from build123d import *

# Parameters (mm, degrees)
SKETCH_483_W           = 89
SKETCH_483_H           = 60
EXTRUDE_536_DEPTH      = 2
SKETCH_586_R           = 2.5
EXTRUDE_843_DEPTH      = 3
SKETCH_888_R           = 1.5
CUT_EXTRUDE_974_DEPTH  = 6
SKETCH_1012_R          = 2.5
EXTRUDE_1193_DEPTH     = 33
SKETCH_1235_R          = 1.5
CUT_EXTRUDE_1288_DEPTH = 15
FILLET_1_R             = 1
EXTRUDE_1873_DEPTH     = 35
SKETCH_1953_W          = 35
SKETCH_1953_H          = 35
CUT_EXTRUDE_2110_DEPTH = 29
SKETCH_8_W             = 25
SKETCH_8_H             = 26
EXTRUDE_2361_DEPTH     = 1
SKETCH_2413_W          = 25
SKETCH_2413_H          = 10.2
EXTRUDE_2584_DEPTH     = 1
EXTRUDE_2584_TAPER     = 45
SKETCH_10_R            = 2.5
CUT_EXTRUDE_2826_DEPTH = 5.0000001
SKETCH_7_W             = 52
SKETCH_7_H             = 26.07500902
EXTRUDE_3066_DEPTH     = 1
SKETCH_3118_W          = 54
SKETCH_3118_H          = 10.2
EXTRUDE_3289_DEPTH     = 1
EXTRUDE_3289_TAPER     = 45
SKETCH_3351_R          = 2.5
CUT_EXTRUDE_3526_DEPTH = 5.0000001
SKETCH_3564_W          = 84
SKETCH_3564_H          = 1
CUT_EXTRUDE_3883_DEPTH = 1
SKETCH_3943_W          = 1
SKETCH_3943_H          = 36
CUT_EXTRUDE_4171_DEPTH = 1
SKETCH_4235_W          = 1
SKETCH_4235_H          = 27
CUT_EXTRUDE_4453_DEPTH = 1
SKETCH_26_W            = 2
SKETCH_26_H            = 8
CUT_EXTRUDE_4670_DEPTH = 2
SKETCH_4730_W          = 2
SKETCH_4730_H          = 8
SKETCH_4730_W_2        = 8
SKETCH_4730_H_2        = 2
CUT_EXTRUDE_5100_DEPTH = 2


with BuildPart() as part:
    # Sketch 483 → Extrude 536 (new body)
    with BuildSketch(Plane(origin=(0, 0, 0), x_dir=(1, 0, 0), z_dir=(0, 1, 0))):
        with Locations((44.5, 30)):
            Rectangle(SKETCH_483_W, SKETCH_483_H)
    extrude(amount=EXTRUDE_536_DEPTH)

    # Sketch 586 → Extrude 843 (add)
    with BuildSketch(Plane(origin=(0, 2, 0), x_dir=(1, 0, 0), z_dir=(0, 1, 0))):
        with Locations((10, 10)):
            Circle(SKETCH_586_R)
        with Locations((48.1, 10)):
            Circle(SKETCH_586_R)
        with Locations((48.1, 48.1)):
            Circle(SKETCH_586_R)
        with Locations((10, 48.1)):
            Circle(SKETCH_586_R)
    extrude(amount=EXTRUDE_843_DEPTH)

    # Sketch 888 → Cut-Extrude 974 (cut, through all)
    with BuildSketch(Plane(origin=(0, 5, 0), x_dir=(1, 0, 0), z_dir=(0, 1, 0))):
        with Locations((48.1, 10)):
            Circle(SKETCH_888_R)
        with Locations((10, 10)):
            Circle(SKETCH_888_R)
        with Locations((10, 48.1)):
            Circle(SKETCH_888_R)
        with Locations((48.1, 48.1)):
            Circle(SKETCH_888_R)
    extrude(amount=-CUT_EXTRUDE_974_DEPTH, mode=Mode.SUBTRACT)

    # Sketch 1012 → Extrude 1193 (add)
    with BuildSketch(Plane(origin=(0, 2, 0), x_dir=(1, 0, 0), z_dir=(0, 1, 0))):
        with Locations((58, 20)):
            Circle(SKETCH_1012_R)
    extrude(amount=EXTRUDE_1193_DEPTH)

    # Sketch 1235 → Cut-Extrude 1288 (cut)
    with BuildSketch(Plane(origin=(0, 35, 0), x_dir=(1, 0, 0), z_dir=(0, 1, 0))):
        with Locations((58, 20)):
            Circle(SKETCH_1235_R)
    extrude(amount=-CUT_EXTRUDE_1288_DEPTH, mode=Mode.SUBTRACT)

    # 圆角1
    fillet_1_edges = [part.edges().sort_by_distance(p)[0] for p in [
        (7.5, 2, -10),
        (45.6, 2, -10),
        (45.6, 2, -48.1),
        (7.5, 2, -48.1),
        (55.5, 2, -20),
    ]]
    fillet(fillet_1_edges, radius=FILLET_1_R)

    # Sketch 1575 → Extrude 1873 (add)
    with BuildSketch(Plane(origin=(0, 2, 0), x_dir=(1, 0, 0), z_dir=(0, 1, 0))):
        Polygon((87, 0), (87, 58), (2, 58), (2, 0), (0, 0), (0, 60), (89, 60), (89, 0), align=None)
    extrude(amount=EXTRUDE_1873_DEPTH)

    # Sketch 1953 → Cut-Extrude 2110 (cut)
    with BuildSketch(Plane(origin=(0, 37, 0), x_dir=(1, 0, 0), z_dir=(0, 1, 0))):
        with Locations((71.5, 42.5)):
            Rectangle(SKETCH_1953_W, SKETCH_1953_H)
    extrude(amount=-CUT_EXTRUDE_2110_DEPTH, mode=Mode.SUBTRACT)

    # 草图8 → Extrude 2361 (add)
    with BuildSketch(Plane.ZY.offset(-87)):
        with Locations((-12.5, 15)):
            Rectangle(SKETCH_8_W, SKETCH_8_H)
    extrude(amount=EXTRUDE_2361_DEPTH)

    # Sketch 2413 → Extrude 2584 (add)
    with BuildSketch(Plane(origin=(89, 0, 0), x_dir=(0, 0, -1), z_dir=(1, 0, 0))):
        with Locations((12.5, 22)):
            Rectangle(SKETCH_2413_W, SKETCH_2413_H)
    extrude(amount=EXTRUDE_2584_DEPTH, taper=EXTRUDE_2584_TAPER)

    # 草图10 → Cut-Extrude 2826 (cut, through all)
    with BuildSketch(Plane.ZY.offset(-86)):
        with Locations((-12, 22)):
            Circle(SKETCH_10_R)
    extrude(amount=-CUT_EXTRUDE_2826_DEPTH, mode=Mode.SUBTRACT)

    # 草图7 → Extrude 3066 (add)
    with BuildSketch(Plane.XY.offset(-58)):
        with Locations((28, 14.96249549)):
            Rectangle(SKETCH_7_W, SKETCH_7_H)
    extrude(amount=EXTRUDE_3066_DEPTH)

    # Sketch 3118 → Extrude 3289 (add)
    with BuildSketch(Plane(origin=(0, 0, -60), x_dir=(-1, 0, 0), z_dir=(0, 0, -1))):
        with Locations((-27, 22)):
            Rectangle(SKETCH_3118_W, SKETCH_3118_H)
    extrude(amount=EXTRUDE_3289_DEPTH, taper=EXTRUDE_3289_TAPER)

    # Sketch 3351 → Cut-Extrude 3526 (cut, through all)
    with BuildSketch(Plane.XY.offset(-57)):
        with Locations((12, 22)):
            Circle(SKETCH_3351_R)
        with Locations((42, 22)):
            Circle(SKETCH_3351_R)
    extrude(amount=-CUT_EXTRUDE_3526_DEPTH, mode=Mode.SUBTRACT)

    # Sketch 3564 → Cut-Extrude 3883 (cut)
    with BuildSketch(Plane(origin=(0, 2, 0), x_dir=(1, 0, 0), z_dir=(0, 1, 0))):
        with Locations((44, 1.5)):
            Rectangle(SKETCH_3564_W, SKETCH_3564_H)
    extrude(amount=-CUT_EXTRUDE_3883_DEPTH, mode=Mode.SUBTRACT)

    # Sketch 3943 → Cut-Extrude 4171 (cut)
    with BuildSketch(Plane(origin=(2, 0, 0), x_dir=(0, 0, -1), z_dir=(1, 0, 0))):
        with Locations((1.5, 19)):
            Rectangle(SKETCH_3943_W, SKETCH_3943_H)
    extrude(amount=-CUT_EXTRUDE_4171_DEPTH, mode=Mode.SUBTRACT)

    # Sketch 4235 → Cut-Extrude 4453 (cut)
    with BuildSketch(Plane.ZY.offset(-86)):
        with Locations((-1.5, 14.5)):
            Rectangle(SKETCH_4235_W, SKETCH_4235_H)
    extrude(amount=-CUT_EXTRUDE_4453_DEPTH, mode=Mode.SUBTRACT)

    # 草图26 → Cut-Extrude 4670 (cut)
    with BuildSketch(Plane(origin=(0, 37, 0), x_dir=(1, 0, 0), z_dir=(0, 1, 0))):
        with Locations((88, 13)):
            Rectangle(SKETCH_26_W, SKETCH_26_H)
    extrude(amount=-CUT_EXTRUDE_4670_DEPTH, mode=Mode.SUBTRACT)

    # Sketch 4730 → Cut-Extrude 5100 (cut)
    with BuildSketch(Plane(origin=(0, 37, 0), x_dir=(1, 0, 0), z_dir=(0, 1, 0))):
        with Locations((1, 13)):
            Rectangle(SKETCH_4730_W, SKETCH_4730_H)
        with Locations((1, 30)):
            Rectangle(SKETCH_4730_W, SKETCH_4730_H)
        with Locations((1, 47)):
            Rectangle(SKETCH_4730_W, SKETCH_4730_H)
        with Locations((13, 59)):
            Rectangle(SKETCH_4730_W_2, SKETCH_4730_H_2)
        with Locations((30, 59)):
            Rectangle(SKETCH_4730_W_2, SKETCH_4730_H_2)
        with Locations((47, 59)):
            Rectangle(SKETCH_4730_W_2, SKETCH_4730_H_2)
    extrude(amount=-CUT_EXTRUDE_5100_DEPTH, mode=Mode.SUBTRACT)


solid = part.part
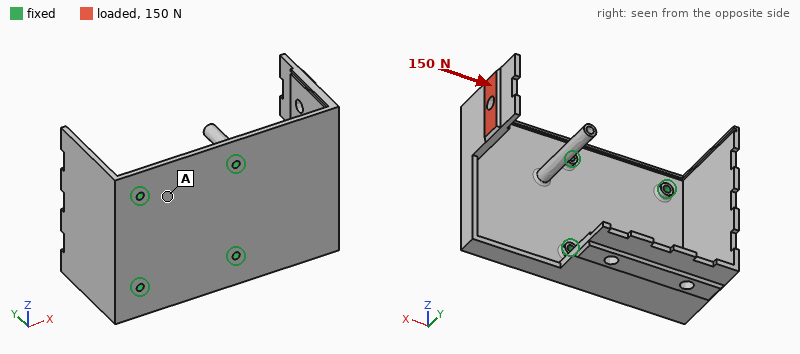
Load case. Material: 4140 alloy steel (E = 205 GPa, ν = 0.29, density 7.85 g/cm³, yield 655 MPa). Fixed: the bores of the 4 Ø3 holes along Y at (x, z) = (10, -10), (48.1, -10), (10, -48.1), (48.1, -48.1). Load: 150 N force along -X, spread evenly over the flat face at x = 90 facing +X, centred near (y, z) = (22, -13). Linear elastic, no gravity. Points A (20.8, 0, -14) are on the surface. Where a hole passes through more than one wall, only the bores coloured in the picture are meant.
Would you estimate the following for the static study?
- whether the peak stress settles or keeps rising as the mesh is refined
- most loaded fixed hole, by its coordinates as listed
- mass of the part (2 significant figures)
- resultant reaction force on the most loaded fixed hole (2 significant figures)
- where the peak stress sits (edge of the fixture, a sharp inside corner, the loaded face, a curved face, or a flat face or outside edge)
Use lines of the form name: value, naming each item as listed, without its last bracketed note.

whether the peak stress settles or keeps rising as the mesh is refined: keeps rising
most loaded fixed hole, by its coordinates as listed: (48.1, -10)
mass of the part: 190 g
resultant reaction force on the most loaded fixed hole: 160 N
where the peak stress sits: a sharp inside corner
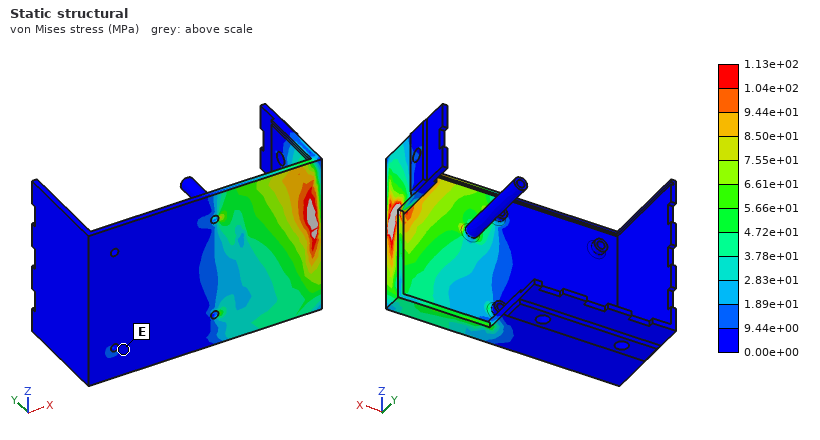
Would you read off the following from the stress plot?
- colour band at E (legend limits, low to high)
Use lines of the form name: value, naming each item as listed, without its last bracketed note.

colour band at E: 0.00e+00 to 9.44e+00 MPa
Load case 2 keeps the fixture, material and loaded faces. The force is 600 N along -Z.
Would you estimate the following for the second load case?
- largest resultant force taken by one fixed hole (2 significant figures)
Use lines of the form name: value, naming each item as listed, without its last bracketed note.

largest resultant force taken by one fixed hole: 780 N
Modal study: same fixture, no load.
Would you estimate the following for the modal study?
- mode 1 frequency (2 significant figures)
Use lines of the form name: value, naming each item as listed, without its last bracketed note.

mode 1 frequency: 550 Hz
